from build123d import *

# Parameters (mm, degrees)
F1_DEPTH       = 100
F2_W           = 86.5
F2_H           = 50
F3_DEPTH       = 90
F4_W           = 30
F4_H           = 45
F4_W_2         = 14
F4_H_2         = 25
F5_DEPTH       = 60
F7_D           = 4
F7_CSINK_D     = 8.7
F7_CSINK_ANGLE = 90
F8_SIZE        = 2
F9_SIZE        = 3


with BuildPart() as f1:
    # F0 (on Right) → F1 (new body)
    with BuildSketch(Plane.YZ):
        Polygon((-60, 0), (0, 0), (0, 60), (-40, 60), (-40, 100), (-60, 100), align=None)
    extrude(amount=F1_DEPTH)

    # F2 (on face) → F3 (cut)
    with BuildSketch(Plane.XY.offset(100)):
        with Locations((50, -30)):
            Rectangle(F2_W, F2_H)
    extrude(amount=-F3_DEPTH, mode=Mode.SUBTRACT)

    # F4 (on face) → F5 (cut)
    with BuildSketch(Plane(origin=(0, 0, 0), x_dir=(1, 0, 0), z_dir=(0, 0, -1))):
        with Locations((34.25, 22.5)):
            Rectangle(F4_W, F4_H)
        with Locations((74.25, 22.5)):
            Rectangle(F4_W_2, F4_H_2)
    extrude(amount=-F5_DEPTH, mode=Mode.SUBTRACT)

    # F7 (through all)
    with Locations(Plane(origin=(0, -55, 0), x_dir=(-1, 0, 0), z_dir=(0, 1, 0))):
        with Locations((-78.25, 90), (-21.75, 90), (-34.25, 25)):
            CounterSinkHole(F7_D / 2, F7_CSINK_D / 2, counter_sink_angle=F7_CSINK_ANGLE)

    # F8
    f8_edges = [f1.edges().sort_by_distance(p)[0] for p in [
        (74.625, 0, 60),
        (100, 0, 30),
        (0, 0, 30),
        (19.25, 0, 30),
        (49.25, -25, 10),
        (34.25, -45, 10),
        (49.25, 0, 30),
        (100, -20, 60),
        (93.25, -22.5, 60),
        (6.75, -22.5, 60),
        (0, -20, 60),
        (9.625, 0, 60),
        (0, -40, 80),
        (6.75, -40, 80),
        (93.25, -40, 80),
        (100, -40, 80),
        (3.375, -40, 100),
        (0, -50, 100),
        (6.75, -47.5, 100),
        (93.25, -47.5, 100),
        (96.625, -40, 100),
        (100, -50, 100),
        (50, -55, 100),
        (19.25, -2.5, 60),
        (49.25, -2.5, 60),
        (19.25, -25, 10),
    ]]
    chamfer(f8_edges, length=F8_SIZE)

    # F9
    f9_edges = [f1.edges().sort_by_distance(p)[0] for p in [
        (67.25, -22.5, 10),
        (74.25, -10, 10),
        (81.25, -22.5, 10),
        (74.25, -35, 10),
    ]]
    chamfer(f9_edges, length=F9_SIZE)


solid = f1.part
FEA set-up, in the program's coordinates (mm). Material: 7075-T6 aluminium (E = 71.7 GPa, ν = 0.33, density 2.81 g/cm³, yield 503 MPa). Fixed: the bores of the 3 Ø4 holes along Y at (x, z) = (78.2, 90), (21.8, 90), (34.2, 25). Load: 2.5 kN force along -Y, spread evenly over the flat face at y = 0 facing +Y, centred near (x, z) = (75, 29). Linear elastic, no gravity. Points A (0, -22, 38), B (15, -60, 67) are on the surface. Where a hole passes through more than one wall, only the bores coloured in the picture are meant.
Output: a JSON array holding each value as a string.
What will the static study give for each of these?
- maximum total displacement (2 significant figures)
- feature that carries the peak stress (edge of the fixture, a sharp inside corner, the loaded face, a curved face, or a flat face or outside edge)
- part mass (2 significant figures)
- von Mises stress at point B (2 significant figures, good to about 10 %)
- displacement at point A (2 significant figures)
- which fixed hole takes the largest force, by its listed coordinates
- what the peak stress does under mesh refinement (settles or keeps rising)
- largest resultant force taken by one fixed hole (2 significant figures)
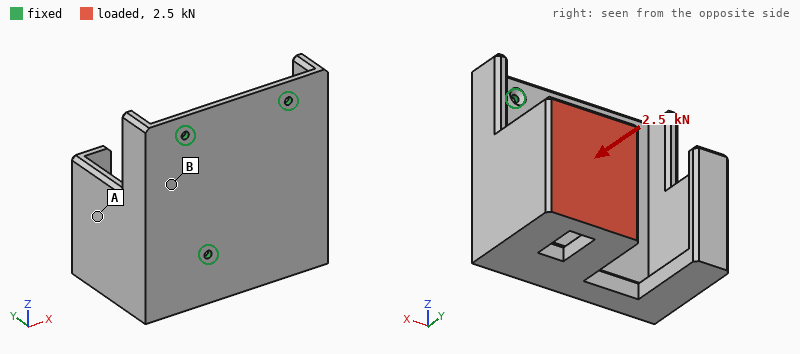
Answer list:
["1.2 mm", "edge of the fixture", "410 g", "34 MPa", "0.40 mm", "(34.2, 25)", "keeps rising", "2.3 kN"]
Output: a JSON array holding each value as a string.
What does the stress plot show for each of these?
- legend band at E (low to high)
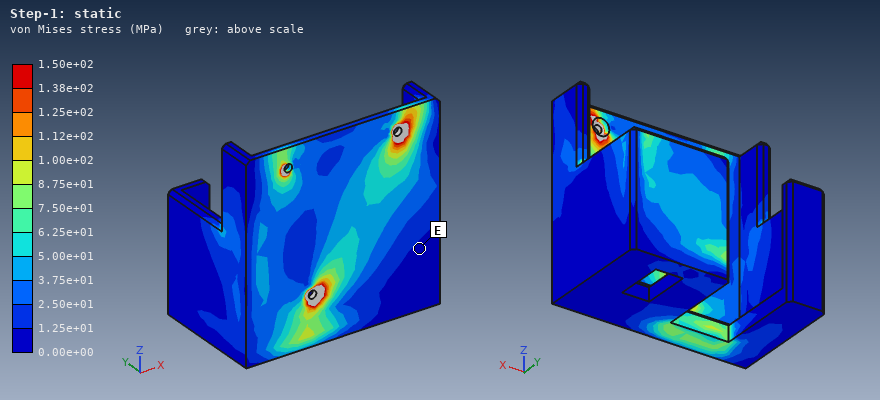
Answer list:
["0.00e+00 to 1.25e+01 MPa"]
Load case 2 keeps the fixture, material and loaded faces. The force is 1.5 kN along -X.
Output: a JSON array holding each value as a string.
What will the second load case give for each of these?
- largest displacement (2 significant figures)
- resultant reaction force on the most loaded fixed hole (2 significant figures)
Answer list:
["1.7 mm", "1.6 kN"]
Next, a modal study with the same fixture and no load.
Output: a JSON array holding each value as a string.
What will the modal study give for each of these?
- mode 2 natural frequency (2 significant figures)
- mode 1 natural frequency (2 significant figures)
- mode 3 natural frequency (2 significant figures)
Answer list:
["1100 Hz", "410 Hz", "1300 Hz"]
